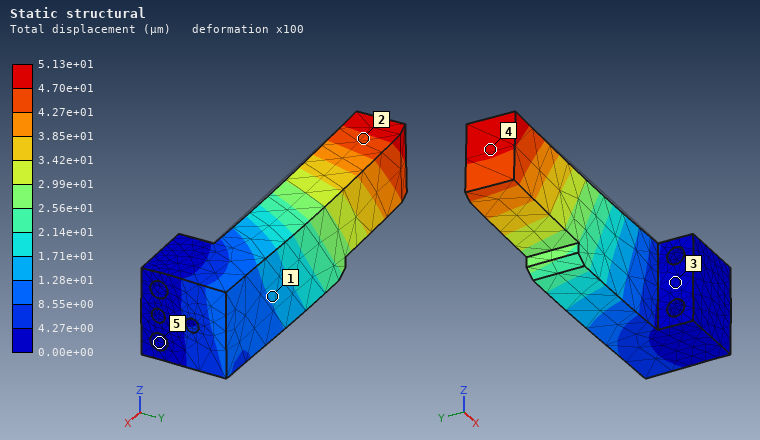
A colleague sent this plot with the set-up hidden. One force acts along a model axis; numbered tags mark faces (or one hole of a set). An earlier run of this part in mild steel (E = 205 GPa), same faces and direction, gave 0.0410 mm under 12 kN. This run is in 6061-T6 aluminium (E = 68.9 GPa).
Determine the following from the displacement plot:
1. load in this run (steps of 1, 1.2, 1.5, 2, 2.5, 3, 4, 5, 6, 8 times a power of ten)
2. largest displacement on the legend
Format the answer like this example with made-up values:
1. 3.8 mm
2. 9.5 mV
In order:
1. 5 kN
2. 5.13e+01 µm
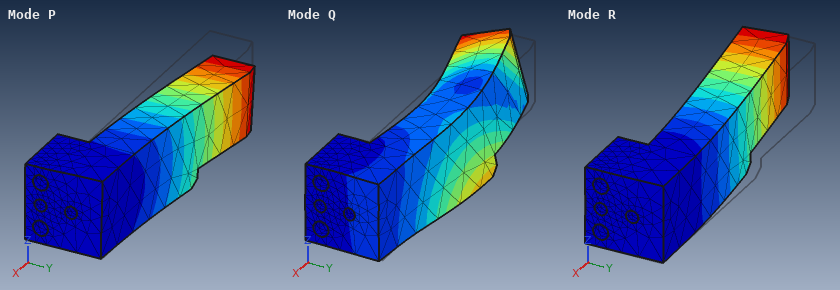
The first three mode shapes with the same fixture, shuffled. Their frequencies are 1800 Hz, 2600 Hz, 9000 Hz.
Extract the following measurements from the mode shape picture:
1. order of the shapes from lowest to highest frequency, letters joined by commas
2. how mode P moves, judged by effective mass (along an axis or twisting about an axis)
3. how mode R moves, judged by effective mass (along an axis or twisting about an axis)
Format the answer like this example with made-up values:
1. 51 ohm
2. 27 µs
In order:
1. R, P, Q
2. along Z
3. along Y
